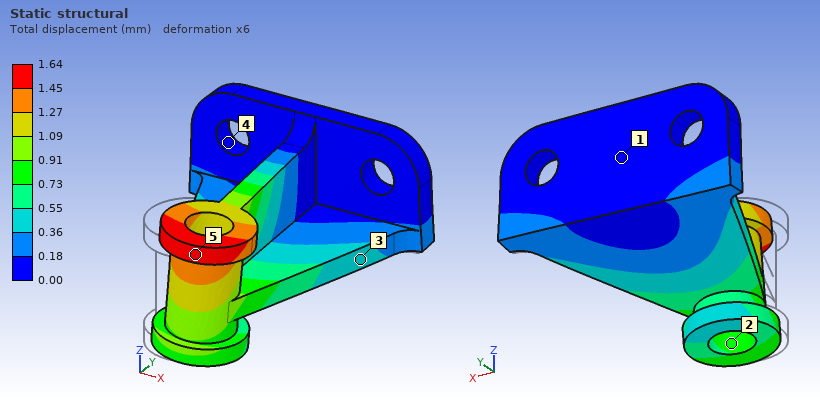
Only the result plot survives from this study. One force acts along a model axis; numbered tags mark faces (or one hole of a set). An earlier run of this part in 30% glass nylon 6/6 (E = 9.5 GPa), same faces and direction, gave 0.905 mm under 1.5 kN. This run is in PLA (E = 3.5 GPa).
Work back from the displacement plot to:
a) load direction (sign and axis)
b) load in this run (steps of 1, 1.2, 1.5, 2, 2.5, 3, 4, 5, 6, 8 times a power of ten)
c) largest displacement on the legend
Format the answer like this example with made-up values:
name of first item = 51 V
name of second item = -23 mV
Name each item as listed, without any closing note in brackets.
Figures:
load direction = +X
load in this run = 1 kN
largest displacement on the legend = 1.64 mm
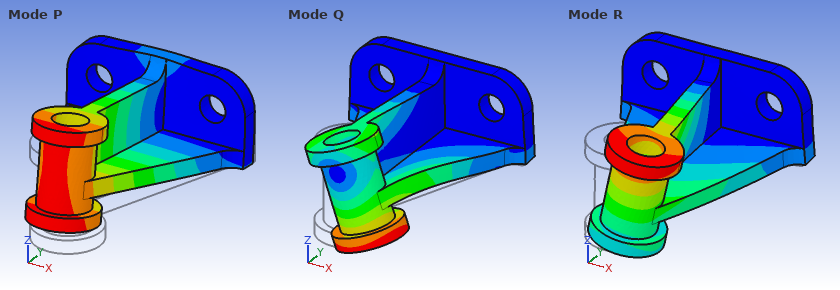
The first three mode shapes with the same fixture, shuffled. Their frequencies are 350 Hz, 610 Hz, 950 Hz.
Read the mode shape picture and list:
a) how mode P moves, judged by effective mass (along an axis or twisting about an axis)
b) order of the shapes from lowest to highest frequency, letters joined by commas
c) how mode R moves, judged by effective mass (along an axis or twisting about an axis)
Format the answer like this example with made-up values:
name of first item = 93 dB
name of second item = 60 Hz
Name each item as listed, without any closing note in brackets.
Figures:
how mode P moves, judged by effective mass = along Z
order of the shapes from lowest to highest frequency, letters joined by commas = P, R, Q
how mode R moves, judged by effective mass = along X
